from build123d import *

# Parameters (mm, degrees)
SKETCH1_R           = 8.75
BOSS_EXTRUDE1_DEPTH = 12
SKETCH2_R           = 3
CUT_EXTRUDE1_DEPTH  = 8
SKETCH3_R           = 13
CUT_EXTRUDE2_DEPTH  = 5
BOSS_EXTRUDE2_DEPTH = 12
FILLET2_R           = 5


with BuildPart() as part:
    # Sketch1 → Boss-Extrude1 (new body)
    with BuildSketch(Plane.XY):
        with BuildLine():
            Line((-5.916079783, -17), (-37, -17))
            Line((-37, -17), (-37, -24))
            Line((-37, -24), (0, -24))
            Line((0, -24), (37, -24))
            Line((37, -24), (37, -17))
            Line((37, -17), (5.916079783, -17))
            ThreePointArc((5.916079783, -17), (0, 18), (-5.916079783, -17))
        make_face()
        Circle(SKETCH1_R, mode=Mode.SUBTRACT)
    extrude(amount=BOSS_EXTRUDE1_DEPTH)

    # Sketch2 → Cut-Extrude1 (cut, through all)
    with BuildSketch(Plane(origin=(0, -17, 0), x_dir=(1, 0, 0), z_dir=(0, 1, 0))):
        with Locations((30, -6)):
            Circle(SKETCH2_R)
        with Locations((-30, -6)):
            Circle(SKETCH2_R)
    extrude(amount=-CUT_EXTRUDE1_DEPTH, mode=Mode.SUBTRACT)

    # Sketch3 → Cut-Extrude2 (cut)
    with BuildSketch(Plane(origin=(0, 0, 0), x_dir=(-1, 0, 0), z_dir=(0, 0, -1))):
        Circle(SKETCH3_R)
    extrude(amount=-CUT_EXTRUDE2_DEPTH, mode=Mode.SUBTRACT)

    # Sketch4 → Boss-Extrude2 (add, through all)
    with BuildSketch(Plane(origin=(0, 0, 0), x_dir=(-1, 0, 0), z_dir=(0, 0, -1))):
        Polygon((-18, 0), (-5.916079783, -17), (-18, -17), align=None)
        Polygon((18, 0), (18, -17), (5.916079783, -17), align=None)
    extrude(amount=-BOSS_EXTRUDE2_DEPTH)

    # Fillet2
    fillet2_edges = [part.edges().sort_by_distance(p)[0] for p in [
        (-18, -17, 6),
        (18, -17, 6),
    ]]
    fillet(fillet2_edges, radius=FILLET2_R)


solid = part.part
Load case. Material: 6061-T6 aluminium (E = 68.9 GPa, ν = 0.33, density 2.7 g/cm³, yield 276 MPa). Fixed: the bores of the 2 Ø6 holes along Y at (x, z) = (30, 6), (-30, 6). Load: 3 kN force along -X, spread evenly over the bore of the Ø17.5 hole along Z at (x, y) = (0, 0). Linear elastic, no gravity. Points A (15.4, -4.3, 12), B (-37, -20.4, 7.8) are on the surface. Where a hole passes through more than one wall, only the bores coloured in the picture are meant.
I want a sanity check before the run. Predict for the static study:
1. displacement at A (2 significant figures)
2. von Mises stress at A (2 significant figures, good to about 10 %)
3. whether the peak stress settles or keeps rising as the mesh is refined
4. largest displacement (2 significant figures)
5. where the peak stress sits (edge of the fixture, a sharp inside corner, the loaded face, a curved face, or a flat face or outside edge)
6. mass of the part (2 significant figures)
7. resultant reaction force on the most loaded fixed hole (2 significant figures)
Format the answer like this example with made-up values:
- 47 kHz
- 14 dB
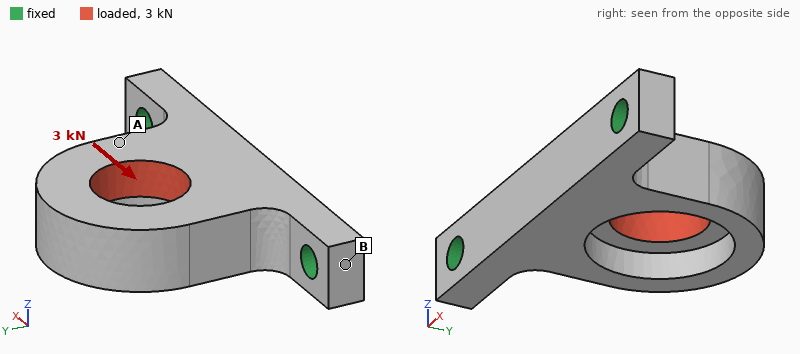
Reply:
- 23 µm
- 25 MPa
- keeps rising
- 47 µm
- edge of the fixture
- 41 g
- 2.0 kN
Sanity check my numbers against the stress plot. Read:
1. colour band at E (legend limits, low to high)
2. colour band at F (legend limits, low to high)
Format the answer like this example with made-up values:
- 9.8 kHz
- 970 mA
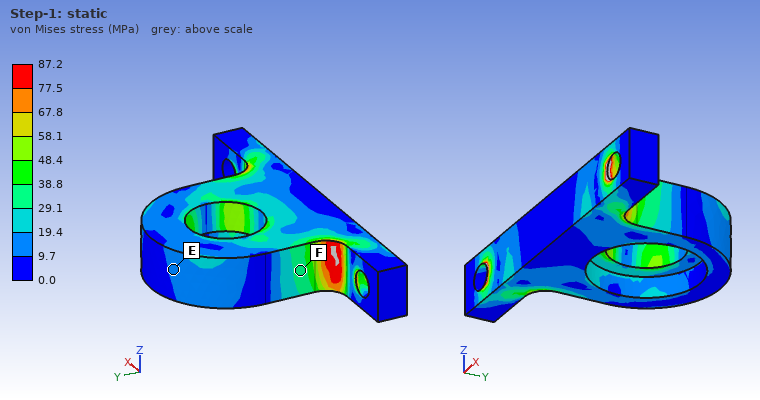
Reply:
- 9.7 to 19.4 MPa
- 29.1 to 38.8 MPa
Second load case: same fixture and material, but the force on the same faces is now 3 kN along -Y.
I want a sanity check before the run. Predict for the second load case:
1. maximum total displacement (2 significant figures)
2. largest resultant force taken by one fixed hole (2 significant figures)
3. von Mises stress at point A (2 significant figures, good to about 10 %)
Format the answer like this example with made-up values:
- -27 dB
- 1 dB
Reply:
- 85 µm
- 1.8 kN
- 23 MPa
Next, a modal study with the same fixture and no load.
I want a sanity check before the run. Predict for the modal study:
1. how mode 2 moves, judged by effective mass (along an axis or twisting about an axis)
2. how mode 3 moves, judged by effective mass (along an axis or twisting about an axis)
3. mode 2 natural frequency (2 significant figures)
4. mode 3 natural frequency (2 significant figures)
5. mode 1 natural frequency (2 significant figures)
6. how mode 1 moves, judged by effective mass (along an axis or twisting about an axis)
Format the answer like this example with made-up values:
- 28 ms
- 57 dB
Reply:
- along X
- along Y
- 9100 Hz
- 10 kHz
- 2900 Hz
- along Z
